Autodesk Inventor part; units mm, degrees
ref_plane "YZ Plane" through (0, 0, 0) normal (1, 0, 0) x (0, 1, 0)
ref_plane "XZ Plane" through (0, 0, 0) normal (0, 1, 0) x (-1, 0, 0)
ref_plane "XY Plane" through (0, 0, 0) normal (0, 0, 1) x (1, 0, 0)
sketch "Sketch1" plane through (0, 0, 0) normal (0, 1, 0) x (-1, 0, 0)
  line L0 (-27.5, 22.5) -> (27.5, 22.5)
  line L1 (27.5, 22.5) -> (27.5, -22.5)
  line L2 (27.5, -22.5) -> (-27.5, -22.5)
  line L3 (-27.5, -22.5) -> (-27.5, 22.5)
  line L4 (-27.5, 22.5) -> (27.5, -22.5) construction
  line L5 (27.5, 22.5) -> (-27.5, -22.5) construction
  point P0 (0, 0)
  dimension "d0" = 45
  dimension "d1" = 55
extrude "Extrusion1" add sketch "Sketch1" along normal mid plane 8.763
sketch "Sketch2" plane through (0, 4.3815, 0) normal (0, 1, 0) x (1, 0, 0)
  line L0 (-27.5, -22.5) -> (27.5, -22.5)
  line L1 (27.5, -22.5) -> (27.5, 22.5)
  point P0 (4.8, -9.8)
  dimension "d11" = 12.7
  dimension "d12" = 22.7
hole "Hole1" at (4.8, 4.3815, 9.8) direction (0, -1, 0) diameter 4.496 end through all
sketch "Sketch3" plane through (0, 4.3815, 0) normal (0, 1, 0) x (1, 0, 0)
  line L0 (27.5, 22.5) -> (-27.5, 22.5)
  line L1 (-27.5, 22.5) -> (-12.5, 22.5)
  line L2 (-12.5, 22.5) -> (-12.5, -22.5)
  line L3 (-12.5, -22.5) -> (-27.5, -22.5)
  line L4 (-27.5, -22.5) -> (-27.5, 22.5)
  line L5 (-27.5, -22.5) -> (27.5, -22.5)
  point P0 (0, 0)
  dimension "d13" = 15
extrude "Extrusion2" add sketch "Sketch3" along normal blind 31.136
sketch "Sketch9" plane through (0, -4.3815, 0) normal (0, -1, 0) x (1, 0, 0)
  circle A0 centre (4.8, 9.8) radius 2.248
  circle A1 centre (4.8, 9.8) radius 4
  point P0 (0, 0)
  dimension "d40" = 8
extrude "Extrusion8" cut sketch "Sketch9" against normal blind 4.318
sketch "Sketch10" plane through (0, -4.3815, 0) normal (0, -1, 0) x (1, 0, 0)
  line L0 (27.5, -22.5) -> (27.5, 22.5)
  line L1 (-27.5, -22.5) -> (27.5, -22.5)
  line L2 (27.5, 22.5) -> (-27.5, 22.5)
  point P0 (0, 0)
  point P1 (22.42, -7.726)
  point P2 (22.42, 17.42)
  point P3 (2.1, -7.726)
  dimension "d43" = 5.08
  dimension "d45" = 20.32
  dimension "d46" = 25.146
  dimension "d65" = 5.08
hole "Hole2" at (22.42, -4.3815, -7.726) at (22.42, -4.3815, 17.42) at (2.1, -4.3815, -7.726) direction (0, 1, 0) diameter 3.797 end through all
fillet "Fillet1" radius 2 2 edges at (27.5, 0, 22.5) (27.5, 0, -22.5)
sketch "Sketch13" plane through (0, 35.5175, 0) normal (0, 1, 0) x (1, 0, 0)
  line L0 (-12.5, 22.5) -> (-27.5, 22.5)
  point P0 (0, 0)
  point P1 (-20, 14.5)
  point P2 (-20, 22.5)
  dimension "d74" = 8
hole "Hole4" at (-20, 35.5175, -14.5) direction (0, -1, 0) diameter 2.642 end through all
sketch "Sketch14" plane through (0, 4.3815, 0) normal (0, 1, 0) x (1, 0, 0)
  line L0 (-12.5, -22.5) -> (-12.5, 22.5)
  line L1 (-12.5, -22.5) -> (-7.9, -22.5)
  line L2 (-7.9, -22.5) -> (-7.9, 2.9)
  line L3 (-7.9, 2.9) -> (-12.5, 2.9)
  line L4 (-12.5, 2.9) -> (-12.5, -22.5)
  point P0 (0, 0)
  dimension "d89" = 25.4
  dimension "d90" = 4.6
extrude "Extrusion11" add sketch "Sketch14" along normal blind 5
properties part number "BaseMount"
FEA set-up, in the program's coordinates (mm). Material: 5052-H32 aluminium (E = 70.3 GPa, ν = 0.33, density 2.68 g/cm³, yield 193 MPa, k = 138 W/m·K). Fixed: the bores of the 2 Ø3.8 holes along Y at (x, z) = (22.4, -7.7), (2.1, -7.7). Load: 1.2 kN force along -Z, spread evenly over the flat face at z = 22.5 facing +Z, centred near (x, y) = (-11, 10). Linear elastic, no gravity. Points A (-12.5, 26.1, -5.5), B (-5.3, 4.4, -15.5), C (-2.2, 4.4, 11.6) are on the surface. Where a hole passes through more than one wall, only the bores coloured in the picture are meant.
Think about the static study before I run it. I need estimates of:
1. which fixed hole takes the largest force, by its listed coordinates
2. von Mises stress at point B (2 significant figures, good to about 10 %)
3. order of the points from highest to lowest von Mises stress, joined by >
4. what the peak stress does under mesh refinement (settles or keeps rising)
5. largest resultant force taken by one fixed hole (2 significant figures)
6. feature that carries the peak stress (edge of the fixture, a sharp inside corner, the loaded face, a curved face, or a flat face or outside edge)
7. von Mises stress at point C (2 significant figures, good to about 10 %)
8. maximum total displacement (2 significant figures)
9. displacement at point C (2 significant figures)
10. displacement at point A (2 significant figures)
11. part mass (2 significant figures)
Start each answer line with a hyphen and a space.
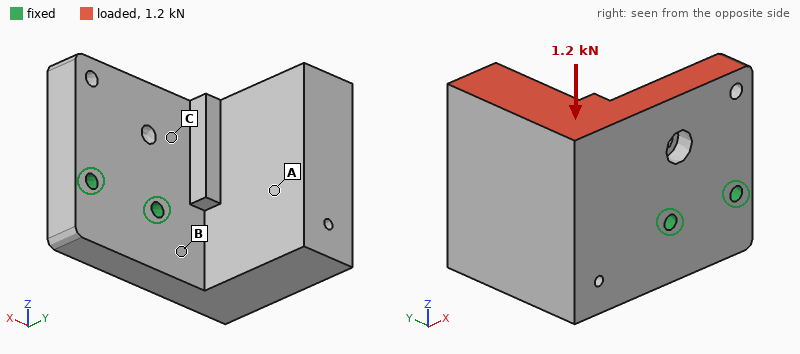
- (2.1, -7.7)
- 19 MPa
- B > C > A
- keeps rising
- 1.8 kN
- edge of the fixture
- 9.7 MPa
- 56 µm
- 17 µm
- 33 µm
- 110 g
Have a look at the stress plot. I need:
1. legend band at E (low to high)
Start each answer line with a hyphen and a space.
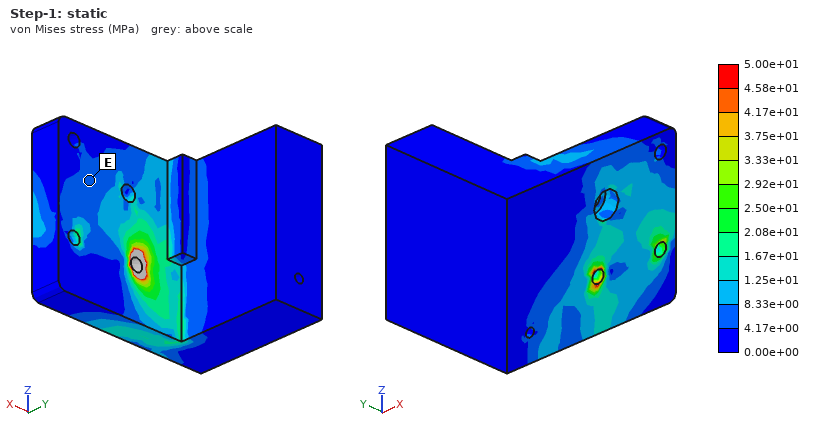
- 4.17e+00 to 8.33e+00 MPa
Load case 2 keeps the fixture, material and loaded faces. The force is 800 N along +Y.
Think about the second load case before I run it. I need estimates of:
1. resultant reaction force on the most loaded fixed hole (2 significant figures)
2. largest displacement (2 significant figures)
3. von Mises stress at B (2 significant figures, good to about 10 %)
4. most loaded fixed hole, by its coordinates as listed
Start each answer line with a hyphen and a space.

- 960 N
- 0.12 mm
- 28 MPa
- (2.1, -7.7)
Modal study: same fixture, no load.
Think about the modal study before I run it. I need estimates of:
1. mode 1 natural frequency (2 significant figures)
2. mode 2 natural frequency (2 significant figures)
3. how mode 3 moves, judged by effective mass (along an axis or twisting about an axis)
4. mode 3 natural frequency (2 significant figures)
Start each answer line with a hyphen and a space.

- 1900 Hz
- 2700 Hz
- along Z
- 6300 Hz
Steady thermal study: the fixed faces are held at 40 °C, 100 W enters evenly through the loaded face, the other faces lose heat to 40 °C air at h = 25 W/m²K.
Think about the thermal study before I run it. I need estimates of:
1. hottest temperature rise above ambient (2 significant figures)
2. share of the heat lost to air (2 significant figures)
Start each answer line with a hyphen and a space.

- 58 K
- 7.9 %
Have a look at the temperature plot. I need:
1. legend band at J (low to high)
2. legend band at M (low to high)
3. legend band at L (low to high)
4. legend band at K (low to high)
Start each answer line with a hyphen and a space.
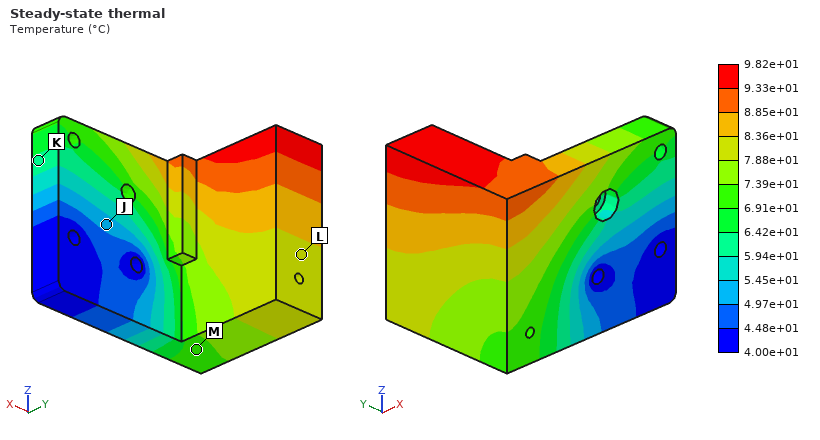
- 4.97e+01 to 5.45e+01 °C
- 6.91e+01 to 7.39e+01 °C
- 7.88e+01 to 8.36e+01 °C
- 5.94e+01 to 6.42e+01 °C
